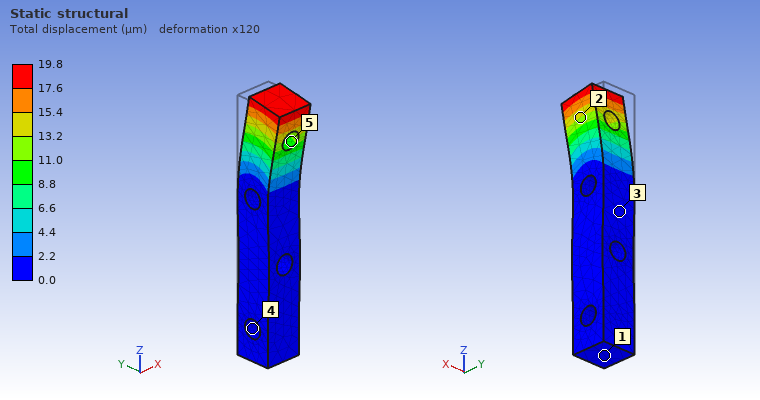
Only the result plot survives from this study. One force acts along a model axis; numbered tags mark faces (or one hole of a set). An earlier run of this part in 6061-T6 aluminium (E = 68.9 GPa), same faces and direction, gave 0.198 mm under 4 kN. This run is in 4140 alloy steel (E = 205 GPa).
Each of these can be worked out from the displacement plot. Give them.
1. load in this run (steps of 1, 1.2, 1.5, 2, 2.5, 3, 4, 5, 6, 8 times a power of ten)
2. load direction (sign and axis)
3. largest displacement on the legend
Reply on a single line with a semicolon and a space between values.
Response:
1.2 kN; -Y; 19.8 µm
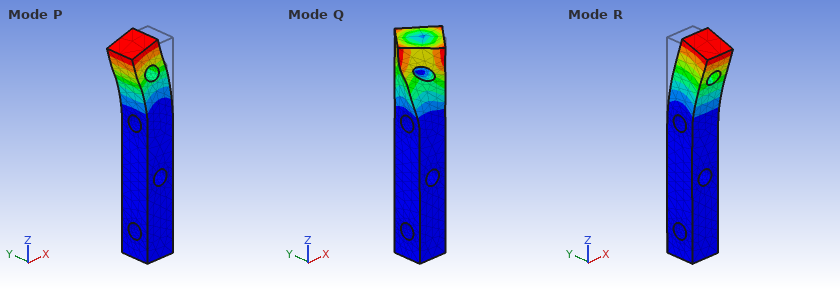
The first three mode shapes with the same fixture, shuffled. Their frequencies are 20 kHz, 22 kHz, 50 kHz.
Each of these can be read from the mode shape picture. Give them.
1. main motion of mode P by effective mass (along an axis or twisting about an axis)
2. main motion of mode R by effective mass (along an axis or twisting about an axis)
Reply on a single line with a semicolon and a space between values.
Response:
along X; along Y
